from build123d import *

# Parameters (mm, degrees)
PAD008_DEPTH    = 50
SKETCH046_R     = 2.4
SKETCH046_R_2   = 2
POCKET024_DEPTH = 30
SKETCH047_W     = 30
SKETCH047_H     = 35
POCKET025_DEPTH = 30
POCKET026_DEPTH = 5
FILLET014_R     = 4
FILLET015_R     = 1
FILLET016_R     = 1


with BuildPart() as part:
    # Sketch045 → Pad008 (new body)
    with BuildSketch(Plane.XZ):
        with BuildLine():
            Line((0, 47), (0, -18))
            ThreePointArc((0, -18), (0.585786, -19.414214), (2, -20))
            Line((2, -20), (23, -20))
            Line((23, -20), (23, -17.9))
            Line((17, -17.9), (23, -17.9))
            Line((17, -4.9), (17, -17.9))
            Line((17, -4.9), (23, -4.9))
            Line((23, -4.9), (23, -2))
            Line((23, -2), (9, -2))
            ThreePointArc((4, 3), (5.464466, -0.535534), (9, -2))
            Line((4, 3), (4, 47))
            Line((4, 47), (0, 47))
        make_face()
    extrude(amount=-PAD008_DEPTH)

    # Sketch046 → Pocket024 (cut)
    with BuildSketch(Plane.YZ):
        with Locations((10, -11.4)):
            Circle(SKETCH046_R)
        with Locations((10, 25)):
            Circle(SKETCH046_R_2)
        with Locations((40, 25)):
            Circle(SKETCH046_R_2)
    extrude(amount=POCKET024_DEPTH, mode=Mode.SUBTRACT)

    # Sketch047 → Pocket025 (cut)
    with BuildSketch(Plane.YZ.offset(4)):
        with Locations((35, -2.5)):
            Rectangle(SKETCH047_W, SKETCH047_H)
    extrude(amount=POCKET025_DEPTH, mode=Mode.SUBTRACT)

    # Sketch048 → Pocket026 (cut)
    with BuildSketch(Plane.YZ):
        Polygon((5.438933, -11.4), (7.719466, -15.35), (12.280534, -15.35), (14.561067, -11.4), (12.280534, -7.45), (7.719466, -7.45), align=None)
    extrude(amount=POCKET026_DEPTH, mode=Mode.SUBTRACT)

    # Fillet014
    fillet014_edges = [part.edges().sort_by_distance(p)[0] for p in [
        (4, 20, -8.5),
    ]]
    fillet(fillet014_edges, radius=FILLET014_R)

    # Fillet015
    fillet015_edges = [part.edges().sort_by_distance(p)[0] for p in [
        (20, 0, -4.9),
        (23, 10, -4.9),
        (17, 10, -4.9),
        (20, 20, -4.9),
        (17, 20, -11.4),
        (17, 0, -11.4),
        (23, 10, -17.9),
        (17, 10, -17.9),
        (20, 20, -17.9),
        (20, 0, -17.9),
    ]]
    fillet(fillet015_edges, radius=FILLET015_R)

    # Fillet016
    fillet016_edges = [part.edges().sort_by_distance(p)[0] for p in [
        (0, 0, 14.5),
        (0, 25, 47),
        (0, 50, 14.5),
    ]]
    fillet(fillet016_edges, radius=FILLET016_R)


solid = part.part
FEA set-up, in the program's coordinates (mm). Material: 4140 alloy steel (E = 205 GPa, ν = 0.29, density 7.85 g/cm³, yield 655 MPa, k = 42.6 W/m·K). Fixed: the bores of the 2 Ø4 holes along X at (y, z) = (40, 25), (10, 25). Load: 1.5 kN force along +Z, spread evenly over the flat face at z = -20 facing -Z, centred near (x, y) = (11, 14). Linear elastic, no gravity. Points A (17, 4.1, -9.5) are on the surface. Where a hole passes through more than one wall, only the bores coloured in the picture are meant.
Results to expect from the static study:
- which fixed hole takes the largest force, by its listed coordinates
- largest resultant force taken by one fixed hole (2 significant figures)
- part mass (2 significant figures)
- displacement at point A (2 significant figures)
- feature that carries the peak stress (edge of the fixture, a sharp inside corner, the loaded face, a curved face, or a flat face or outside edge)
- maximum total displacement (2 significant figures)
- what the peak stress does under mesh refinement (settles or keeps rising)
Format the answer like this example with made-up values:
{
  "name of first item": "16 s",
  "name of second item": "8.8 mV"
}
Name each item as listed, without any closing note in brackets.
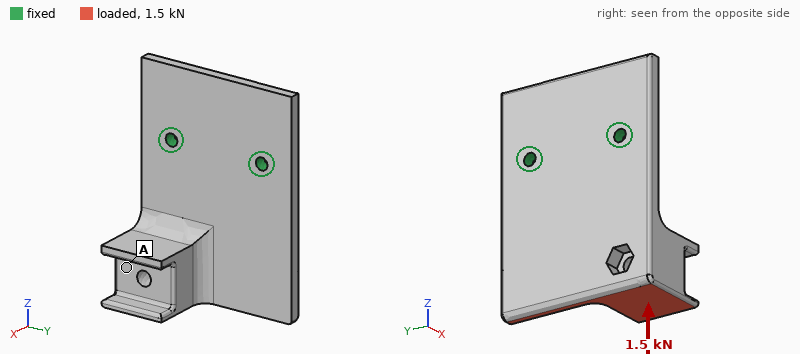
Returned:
{
  "which fixed hole takes the largest force, by its listed coordinates": "(10, 25)",
  "largest resultant force taken by one fixed hole": "1.3 kN",
  "part mass": "140 g",
  "displacement at point A": "0.20 mm",
  "feature that carries the peak stress": "edge of the fixture",
  "maximum total displacement": "0.30 mm",
  "what the peak stress does under mesh refinement": "keeps rising"
}
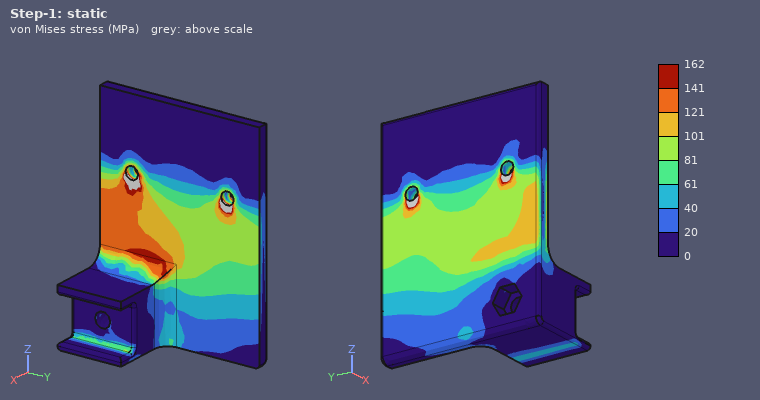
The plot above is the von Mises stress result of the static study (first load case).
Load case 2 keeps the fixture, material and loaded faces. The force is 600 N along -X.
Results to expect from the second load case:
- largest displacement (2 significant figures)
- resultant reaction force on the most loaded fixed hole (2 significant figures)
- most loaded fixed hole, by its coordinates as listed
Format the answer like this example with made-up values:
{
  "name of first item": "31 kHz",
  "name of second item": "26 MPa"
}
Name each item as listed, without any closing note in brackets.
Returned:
{
  "largest displacement": "0.43 mm",
  "resultant reaction force on the most loaded fixed hole": "490 N",
  "most loaded fixed hole, by its coordinates as listed": "(10, 25)"
}
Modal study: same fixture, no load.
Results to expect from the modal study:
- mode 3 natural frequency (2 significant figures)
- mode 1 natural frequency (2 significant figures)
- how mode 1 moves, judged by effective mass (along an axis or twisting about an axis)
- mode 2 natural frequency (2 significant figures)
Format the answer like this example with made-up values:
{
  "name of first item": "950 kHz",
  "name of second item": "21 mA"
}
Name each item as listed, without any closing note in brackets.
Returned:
{
  "mode 3 natural frequency": "5700 Hz",
  "mode 1 natural frequency": "1000 Hz",
  "how mode 1 moves, judged by effective mass": "along X",
  "mode 2 natural frequency": "2800 Hz"
}
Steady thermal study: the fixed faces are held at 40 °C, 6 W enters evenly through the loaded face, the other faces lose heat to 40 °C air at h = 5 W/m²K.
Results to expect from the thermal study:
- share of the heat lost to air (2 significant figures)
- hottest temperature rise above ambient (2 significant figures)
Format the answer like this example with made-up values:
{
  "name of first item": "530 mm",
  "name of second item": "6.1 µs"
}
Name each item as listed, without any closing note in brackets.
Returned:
{
  "share of the heat lost to air": "9.7 %",
  "hottest temperature rise above ambient": "35 K"
}
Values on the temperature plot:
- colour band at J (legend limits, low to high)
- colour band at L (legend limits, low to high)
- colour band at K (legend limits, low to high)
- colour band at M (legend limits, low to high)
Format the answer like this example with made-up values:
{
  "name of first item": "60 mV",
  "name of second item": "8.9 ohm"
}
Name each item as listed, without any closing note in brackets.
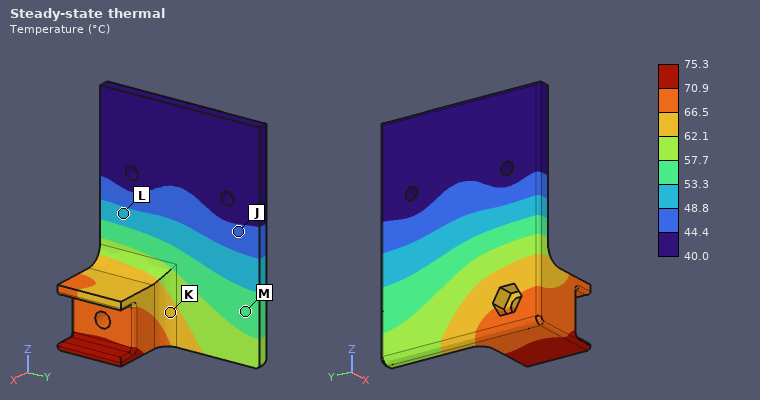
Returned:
{
  "colour band at J": "44.4 to 48.8 °C",
  "colour band at L": "48.8 to 53.3 °C",
  "colour band at K": "62.1 to 66.5 °C",
  "colour band at M": "53.3 to 57.7 °C"
}
